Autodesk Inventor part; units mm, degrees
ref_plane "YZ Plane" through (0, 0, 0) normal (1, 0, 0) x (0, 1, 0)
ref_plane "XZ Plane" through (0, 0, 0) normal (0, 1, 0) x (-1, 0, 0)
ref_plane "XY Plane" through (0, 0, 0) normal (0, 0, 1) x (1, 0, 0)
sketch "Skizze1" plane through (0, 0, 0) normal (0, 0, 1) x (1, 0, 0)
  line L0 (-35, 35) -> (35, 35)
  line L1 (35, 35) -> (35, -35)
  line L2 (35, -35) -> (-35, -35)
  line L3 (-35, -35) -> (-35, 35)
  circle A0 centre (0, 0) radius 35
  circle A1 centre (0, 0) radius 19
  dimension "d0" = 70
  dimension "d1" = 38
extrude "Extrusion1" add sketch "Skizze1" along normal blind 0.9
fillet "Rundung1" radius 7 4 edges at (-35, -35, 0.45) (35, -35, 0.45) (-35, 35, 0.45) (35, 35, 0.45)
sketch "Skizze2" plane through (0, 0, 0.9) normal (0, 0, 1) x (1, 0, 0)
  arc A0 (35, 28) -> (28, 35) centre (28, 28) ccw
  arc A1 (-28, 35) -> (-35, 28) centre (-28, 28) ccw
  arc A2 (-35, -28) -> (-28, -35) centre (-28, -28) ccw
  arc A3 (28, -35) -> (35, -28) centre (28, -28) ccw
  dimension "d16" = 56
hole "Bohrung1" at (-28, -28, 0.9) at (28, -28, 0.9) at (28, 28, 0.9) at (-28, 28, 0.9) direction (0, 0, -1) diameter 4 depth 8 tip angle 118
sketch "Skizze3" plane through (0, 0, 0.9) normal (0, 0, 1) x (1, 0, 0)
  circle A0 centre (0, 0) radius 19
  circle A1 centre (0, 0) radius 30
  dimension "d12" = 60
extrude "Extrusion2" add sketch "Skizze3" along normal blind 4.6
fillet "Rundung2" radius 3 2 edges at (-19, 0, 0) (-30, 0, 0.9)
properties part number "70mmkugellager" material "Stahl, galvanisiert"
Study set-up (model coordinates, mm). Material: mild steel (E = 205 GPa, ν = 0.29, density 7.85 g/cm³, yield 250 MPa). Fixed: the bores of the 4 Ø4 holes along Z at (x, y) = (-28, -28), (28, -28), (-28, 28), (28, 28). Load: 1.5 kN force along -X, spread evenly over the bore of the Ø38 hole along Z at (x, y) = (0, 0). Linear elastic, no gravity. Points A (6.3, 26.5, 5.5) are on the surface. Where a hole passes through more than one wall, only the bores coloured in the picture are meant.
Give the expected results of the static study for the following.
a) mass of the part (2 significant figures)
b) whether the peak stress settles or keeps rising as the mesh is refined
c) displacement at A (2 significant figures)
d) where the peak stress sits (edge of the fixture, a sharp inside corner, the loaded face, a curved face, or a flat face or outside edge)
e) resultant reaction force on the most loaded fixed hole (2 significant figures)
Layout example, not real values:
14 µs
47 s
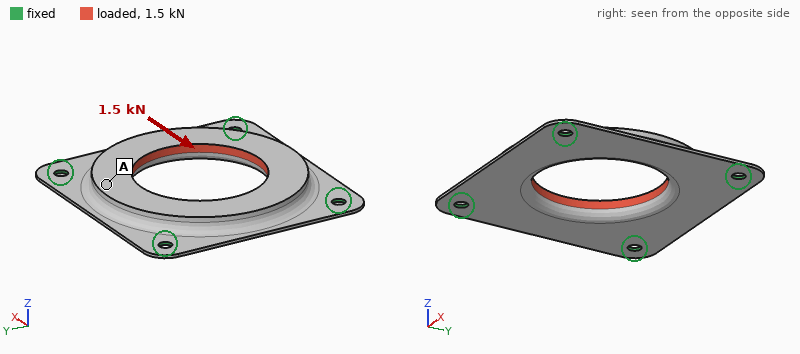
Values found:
88 g
keeps rising
4.2 µm
edge of the fixture
390 N
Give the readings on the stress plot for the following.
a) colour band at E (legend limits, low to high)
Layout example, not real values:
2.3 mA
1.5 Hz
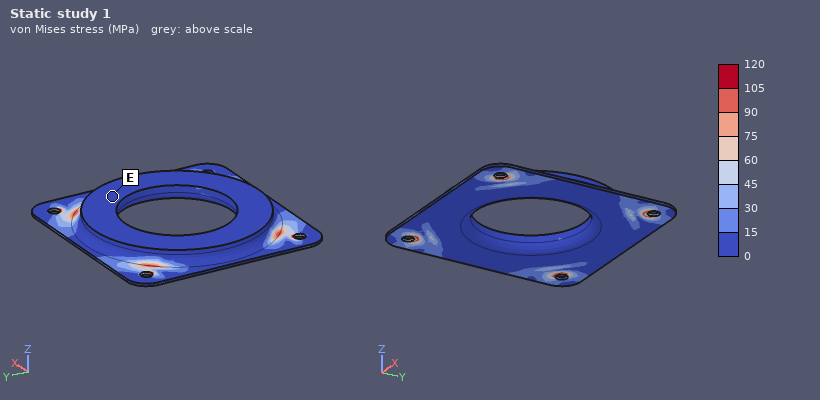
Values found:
0 to 15 MPa
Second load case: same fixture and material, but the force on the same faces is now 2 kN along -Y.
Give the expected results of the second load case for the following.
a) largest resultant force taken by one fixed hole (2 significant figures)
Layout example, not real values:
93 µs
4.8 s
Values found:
530 N
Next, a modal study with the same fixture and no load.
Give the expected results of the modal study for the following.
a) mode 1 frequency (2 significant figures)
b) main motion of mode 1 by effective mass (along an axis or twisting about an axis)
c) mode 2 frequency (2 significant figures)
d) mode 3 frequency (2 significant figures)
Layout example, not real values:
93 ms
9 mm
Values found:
2400 Hz
along Z
3200 Hz
3200 Hz
